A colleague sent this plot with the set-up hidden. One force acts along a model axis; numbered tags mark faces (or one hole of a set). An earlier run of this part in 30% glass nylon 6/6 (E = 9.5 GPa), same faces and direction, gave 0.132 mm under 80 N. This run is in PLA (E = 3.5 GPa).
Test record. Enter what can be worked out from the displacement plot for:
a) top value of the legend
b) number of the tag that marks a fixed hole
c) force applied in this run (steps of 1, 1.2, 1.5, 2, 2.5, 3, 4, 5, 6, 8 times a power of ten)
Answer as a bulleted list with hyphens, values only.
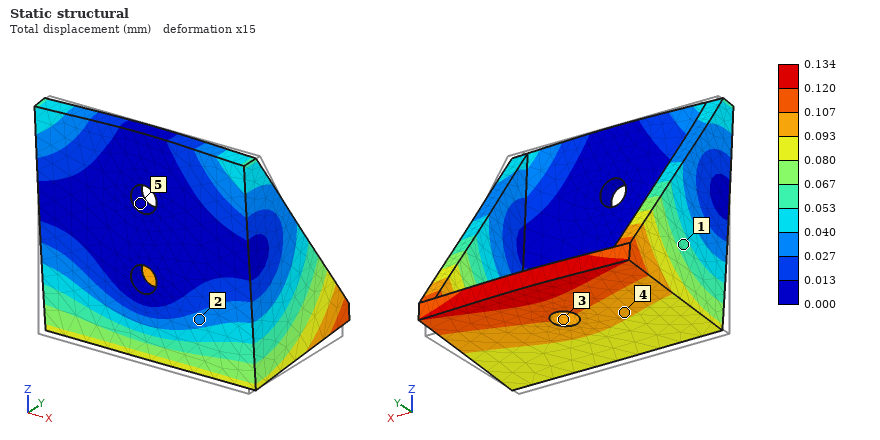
- 0.134 mm
- 5
- 30 N
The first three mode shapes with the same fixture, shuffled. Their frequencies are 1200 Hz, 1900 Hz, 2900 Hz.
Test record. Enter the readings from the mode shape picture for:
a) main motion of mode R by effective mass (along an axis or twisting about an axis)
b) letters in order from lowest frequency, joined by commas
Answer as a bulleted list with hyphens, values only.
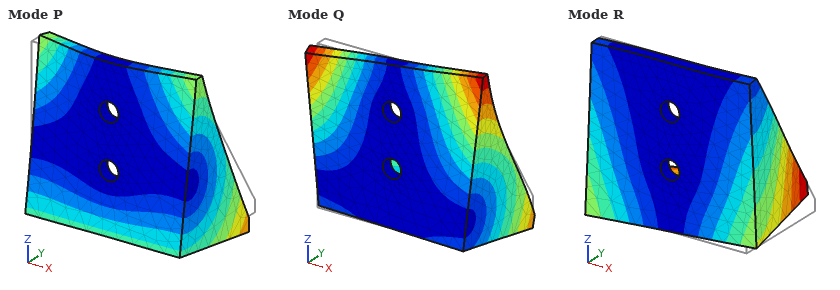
- along X
- R, P, Q
